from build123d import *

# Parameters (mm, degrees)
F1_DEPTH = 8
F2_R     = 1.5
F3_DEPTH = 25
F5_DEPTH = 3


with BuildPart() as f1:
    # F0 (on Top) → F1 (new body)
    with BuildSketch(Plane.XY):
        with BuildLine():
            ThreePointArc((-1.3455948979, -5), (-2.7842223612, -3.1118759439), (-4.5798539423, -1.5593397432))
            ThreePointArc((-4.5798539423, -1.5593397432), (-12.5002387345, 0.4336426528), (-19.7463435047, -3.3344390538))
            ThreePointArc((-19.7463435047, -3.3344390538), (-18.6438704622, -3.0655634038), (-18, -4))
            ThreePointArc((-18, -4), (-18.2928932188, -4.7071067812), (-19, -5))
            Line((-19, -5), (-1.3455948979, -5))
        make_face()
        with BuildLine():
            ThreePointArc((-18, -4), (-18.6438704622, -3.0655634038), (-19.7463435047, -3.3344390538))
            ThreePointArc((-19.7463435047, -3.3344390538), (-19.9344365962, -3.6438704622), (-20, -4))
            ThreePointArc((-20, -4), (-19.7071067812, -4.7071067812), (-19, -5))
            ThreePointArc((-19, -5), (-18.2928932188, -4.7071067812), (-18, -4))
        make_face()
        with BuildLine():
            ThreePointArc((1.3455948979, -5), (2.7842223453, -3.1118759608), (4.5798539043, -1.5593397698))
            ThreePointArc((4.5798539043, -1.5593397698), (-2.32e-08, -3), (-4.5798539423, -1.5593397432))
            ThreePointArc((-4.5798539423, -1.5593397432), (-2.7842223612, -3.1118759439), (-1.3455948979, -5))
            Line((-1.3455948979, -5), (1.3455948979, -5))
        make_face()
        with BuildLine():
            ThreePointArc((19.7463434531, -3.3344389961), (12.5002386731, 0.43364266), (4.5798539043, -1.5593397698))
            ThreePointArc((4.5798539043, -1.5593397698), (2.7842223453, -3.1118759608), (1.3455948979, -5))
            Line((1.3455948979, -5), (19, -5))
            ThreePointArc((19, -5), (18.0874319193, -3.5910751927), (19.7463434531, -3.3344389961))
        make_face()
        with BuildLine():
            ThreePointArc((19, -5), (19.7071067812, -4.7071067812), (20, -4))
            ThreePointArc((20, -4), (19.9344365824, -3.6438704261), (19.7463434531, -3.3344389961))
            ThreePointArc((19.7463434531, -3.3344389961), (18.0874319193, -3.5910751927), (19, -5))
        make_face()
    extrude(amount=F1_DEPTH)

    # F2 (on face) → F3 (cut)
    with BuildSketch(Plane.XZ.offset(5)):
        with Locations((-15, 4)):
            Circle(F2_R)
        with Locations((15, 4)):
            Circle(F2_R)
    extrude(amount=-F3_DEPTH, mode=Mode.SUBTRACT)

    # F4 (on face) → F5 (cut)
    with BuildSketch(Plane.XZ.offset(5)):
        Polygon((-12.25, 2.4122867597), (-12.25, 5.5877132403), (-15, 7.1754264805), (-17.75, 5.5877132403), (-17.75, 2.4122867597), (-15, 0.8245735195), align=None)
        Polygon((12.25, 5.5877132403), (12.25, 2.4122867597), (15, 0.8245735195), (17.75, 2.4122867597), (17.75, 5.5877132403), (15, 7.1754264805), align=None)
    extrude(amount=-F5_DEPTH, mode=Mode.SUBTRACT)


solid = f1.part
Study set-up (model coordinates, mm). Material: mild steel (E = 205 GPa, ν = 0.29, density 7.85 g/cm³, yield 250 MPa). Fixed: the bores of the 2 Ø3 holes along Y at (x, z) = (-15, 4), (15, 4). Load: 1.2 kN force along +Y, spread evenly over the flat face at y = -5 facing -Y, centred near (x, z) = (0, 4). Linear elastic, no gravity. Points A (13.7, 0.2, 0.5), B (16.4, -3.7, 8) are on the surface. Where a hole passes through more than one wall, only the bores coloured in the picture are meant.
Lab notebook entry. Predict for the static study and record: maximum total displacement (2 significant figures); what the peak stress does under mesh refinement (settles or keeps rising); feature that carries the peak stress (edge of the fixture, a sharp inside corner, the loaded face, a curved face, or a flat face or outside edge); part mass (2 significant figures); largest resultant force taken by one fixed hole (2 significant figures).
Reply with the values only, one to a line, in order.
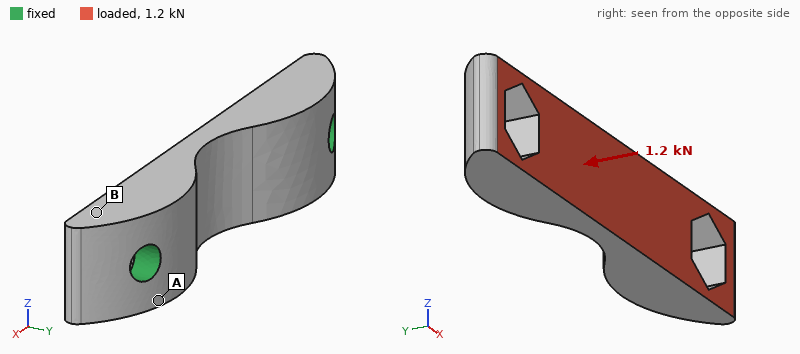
11 µm
keeps rising
edge of the fixture
8.7 g
930 N
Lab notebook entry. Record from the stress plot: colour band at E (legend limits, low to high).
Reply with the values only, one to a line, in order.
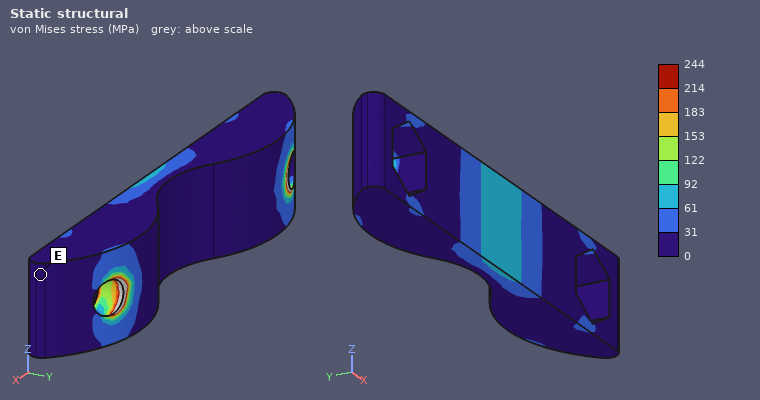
0 to 31 MPa
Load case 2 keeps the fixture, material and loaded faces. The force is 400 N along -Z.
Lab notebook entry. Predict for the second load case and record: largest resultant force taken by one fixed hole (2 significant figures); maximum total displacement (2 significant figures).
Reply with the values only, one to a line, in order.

200 N
6.1 µm
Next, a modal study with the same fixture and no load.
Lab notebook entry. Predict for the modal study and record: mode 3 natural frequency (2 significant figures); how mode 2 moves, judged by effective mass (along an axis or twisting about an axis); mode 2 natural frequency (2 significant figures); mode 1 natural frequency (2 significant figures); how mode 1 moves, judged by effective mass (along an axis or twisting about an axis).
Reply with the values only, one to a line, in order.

38 kHz
along Y
24 kHz
22 kHz
along Z
